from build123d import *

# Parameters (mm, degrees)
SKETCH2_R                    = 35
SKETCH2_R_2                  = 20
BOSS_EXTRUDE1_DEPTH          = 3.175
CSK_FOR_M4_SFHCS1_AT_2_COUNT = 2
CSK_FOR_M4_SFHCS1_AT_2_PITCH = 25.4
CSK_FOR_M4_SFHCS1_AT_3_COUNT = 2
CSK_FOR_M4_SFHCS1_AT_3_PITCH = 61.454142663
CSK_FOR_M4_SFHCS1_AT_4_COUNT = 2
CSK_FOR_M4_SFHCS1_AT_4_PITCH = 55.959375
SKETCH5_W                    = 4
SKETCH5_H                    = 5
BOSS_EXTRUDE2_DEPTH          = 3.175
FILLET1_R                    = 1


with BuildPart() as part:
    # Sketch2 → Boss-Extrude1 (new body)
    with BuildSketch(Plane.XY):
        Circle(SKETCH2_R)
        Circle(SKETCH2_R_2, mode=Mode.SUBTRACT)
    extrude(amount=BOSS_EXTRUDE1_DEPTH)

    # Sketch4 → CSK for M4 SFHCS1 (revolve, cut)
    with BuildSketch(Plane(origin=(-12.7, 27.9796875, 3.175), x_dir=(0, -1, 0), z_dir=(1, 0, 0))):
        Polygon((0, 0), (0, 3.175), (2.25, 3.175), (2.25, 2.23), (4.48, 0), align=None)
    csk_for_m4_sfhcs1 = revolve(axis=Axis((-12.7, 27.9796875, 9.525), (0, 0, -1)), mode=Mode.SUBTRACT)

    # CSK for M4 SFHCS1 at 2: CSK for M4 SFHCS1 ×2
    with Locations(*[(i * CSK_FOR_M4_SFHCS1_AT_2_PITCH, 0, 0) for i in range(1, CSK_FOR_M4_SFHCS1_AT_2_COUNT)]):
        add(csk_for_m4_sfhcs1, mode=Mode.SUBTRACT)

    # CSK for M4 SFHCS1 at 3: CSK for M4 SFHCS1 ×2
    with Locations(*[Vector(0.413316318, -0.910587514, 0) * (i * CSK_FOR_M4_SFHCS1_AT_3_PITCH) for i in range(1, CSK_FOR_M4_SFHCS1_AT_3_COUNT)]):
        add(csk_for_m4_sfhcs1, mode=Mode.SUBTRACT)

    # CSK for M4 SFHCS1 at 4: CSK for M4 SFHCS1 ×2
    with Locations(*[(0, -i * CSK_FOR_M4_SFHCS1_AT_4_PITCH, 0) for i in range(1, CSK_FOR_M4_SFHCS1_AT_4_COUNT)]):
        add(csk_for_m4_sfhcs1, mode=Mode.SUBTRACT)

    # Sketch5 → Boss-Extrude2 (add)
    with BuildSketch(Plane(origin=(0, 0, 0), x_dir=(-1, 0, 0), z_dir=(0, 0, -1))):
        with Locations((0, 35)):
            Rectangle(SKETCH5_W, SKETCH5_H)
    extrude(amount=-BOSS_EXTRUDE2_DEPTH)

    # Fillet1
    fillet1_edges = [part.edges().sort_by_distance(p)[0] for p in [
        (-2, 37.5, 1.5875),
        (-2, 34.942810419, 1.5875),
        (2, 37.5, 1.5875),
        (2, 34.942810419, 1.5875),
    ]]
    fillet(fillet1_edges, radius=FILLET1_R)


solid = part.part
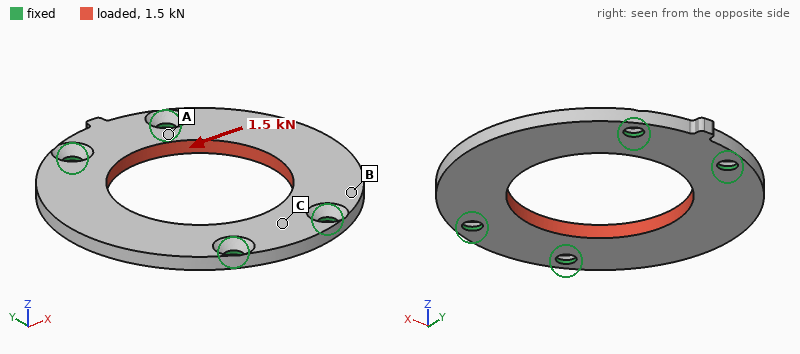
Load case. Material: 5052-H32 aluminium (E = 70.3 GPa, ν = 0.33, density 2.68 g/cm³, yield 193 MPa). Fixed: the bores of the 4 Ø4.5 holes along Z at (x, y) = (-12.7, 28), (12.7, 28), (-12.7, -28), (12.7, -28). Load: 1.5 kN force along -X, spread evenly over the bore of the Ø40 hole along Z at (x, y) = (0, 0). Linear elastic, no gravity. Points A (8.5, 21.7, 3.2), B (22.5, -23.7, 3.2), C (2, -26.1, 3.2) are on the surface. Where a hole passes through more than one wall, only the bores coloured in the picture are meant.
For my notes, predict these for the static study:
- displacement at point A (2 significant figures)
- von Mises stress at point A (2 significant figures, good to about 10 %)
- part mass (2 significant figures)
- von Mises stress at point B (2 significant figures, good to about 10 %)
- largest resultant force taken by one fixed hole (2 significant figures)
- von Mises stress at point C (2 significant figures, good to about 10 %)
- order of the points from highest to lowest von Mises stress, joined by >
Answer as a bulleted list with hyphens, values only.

- 2.5 µm
- 14 MPa
- 21 g
- 3.9 MPa
- 380 N
- 8.7 MPa
- A > C > B
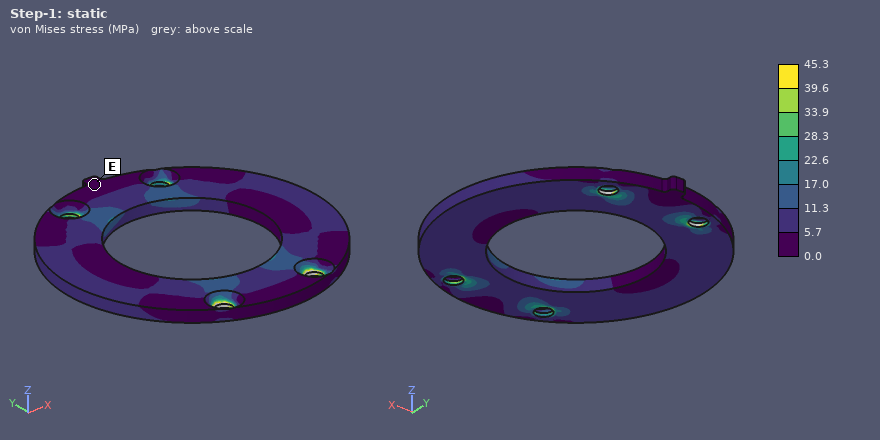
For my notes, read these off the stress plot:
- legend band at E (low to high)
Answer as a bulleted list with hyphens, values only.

- 0.0 to 5.7 MPa
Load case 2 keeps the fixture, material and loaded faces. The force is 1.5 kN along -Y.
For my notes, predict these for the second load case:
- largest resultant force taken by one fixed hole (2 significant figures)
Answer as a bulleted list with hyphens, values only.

- 380 N
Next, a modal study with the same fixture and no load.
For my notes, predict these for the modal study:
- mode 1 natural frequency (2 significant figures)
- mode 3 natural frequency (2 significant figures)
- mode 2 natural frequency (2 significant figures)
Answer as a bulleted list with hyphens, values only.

- 2800 Hz
- 8000 Hz
- 2800 Hz
